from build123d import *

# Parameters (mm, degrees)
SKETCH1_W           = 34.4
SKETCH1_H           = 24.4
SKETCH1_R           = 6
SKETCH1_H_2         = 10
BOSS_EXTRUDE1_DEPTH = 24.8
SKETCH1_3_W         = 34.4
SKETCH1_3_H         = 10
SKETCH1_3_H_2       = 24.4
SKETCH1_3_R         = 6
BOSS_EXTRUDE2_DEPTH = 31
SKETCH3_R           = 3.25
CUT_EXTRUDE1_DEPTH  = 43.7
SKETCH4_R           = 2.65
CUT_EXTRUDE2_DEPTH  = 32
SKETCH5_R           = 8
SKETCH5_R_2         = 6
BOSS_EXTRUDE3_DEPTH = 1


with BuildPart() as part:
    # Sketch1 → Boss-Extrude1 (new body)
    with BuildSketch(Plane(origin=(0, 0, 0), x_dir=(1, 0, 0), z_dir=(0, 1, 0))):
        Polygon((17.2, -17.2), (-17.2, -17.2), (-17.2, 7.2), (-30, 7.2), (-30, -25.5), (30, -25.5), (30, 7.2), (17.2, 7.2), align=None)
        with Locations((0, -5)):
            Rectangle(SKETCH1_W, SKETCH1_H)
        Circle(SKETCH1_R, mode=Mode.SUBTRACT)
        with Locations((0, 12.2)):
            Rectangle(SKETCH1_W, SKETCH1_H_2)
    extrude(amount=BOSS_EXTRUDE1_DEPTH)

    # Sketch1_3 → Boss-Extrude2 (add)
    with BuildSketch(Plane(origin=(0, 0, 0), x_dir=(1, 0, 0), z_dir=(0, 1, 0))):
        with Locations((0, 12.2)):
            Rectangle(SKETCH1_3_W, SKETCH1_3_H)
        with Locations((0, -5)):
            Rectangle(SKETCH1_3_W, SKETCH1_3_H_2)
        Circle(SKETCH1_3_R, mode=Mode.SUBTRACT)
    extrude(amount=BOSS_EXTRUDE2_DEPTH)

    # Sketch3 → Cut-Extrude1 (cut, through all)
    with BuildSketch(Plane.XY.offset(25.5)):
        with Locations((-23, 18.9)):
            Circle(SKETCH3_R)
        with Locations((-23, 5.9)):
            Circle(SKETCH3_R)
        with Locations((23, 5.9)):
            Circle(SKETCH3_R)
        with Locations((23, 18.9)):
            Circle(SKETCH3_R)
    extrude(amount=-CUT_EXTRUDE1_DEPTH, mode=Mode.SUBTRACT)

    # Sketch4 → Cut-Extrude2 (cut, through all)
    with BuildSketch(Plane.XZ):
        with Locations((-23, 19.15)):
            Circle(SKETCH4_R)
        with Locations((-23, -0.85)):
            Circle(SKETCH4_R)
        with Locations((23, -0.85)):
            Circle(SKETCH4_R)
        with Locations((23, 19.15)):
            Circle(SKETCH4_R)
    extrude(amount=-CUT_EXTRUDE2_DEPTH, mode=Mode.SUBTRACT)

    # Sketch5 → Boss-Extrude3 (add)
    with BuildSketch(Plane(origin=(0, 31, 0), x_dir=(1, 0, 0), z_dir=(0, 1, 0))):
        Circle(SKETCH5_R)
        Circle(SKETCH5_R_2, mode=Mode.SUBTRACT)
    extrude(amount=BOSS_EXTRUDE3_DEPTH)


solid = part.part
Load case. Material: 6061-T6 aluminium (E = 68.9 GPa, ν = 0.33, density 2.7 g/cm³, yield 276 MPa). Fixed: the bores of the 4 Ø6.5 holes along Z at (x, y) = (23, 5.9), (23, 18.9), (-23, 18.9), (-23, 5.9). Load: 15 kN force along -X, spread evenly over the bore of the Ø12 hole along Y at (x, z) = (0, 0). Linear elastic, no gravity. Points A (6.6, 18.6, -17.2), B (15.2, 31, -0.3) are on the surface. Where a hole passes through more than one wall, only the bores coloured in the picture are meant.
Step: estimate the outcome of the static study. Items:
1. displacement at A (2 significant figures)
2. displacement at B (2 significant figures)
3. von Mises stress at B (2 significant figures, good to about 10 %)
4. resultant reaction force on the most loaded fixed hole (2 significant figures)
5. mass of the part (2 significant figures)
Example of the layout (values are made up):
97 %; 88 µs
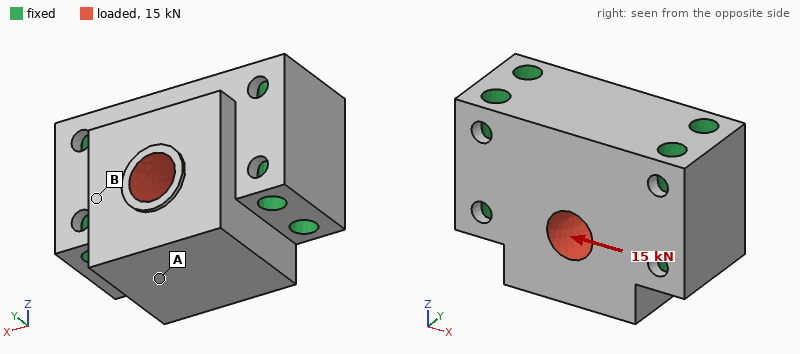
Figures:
3.1 µm; 3.9 µm; 8.7 MPa; 4.4 kN; 150 g
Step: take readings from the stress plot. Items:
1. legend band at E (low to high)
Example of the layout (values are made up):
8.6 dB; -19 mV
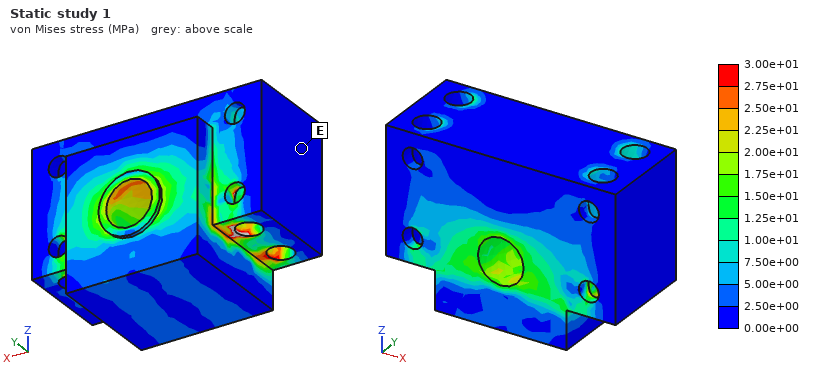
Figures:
0.00e+00 to 2.50e+00 MPa
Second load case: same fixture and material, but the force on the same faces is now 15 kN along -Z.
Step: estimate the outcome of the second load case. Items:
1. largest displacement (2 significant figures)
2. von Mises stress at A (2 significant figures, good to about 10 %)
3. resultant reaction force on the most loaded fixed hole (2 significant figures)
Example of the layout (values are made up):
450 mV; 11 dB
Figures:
11 µm; 11 MPa; 4.7 kN
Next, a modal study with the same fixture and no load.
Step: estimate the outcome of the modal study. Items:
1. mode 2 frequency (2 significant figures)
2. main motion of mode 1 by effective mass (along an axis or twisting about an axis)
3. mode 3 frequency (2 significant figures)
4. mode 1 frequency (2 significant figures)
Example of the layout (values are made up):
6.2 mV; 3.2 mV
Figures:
29 kHz; along Y; 31 kHz; 20 kHz
